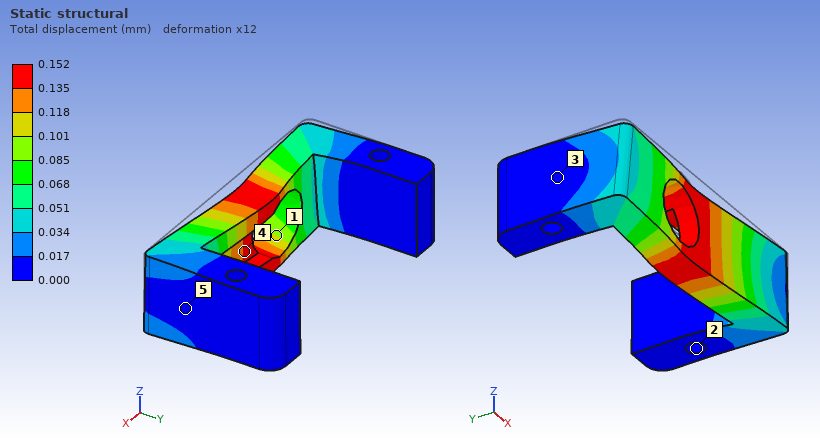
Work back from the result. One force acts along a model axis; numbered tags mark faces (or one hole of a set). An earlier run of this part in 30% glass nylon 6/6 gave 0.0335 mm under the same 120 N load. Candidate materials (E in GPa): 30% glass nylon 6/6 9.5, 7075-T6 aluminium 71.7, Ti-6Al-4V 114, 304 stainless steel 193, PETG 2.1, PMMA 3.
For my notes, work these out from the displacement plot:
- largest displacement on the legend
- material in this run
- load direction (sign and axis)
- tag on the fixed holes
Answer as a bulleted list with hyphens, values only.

- 0.152 mm
- PETG
- -Z
- 2
